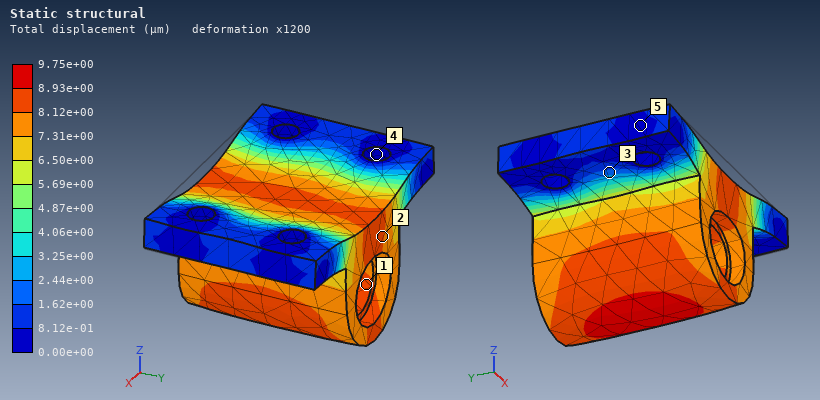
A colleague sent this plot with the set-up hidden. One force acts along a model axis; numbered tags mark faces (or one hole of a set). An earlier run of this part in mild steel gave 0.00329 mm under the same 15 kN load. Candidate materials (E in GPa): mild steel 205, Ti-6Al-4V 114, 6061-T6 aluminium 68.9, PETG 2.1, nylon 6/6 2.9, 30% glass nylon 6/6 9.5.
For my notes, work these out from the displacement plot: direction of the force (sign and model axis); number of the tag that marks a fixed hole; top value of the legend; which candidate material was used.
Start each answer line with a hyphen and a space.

- -Z
- 4
- 9.75e+00 µm
- 6061-T6 aluminium
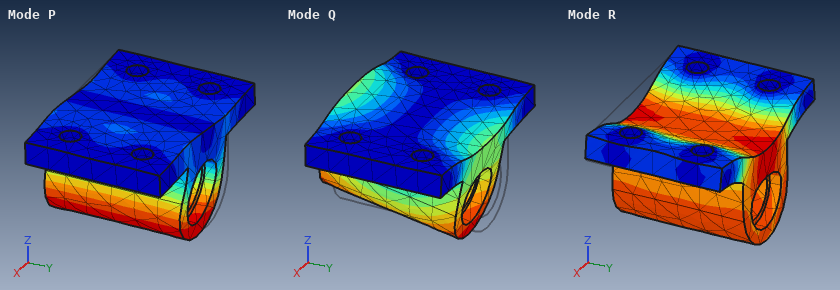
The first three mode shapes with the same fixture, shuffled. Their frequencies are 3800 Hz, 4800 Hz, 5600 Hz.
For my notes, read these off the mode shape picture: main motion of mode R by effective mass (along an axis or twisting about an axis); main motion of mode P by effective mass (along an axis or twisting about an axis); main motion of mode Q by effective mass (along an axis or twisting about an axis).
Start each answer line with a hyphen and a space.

- along Z
- along X
- along Y
